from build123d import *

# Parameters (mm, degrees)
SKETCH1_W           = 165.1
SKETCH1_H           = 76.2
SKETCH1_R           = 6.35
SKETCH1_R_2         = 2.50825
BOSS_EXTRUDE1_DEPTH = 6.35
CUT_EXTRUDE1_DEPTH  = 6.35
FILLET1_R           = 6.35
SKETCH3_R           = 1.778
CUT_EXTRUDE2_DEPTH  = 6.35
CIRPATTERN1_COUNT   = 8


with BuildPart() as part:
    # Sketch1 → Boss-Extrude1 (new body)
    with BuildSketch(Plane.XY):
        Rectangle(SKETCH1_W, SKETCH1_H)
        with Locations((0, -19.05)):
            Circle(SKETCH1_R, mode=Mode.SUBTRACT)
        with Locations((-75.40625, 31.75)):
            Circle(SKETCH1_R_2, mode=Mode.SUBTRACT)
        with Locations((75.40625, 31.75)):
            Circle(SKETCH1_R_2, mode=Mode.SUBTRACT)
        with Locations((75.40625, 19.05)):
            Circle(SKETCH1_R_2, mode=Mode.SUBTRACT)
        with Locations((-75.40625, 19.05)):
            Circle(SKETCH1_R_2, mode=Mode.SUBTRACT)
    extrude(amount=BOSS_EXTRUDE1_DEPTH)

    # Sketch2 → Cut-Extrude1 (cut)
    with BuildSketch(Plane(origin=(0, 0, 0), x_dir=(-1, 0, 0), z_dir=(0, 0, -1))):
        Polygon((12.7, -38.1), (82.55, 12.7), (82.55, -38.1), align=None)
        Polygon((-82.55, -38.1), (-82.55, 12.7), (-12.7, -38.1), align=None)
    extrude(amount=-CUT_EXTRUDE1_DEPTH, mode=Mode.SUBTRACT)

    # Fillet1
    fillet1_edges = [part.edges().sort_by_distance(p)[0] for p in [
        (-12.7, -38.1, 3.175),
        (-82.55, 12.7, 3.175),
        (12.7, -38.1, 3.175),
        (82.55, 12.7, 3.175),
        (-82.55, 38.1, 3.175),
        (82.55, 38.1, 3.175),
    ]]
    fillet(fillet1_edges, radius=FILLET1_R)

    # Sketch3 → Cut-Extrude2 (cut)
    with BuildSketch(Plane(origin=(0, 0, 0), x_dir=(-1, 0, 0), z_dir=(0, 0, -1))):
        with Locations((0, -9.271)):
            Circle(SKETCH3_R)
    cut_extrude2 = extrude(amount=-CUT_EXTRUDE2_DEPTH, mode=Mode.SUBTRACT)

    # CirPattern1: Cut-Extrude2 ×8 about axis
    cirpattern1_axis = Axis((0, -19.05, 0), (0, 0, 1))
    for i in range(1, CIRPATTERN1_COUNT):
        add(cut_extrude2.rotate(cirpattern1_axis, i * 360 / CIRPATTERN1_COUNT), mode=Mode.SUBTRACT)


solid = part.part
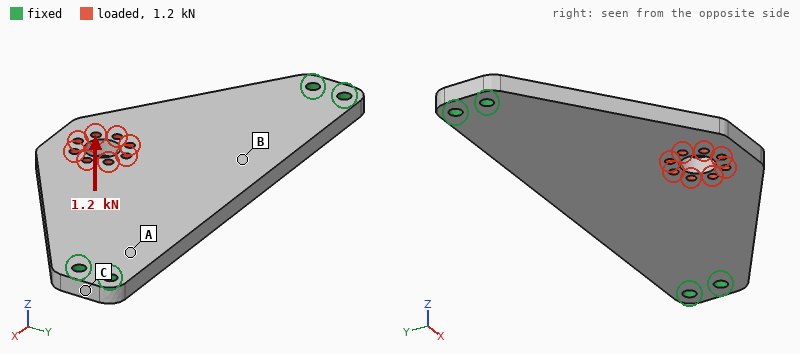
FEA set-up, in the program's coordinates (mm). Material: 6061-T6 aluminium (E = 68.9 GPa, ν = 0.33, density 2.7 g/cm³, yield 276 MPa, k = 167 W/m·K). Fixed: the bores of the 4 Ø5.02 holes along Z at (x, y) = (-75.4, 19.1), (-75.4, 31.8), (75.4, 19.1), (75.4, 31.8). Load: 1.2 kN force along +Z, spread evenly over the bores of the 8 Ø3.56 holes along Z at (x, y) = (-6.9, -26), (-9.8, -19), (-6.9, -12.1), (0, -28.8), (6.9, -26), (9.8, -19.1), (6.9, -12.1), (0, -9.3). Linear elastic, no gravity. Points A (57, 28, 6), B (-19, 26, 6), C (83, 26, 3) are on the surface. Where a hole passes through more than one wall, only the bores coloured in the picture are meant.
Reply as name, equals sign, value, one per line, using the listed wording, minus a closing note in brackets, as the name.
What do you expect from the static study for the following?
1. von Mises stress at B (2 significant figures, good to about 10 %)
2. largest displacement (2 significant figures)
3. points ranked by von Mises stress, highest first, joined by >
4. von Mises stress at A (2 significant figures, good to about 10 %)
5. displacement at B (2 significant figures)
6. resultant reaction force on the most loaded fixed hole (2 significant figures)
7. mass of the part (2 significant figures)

von Mises stress at B = 36 MPa
largest displacement = 1.1 mm
points ranked by von Mises stress, highest first, joined by > = A > B > C
von Mises stress at A = 75 MPa
displacement at B = 0.18 mm
resultant reaction force on the most loaded fixed hole = 1.4 kN
mass of the part = 150 g
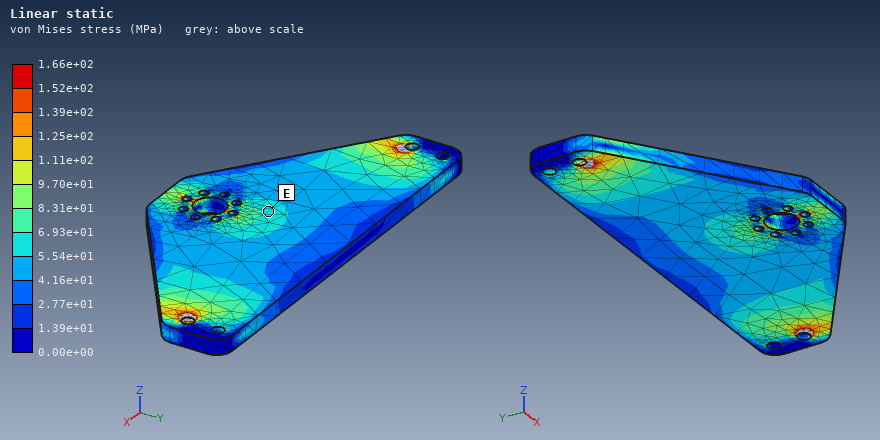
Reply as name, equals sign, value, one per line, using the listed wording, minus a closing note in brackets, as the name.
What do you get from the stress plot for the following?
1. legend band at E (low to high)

legend band at E = 5.54e+01 to 6.93e+01 MPa
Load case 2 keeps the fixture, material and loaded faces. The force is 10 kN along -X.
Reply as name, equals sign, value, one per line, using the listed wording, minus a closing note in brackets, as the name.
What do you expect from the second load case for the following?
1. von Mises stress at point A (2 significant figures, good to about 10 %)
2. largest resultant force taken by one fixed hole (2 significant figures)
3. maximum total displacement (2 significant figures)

von Mises stress at point A = 18 MPa
largest resultant force taken by one fixed hole = 3.5 kN
maximum total displacement = 48 µm
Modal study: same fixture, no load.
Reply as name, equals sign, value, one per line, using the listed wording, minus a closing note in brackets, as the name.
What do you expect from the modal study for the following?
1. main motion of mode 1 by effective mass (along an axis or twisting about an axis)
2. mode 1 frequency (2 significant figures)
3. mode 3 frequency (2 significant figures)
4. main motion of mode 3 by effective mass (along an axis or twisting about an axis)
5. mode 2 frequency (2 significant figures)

main motion of mode 1 by effective mass = along Z
mode 1 frequency = 940 Hz
mode 3 frequency = 3000 Hz
main motion of mode 3 by effective mass = twisting about Y
mode 2 frequency = 1900 Hz
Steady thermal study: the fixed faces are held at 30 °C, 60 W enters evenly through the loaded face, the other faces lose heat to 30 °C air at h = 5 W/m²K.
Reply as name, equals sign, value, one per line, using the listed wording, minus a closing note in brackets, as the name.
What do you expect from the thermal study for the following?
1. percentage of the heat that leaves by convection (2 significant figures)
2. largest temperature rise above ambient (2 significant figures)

percentage of the heat that leaves by convection = 4.8 %
largest temperature rise above ambient = 62 K
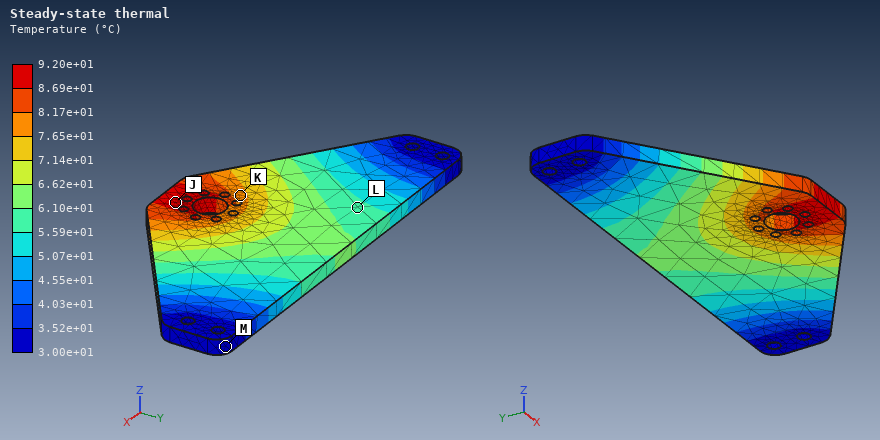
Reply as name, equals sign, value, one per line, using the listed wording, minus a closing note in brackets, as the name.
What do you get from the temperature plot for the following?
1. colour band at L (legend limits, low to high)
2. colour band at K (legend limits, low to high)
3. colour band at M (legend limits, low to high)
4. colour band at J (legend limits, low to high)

colour band at L = 5.59e+01 to 6.10e+01 °C
colour band at K = 7.65e+01 to 8.17e+01 °C
colour band at M = 3.00e+01 to 3.52e+01 °C
colour band at J = 8.69e+01 to 9.20e+01 °C
